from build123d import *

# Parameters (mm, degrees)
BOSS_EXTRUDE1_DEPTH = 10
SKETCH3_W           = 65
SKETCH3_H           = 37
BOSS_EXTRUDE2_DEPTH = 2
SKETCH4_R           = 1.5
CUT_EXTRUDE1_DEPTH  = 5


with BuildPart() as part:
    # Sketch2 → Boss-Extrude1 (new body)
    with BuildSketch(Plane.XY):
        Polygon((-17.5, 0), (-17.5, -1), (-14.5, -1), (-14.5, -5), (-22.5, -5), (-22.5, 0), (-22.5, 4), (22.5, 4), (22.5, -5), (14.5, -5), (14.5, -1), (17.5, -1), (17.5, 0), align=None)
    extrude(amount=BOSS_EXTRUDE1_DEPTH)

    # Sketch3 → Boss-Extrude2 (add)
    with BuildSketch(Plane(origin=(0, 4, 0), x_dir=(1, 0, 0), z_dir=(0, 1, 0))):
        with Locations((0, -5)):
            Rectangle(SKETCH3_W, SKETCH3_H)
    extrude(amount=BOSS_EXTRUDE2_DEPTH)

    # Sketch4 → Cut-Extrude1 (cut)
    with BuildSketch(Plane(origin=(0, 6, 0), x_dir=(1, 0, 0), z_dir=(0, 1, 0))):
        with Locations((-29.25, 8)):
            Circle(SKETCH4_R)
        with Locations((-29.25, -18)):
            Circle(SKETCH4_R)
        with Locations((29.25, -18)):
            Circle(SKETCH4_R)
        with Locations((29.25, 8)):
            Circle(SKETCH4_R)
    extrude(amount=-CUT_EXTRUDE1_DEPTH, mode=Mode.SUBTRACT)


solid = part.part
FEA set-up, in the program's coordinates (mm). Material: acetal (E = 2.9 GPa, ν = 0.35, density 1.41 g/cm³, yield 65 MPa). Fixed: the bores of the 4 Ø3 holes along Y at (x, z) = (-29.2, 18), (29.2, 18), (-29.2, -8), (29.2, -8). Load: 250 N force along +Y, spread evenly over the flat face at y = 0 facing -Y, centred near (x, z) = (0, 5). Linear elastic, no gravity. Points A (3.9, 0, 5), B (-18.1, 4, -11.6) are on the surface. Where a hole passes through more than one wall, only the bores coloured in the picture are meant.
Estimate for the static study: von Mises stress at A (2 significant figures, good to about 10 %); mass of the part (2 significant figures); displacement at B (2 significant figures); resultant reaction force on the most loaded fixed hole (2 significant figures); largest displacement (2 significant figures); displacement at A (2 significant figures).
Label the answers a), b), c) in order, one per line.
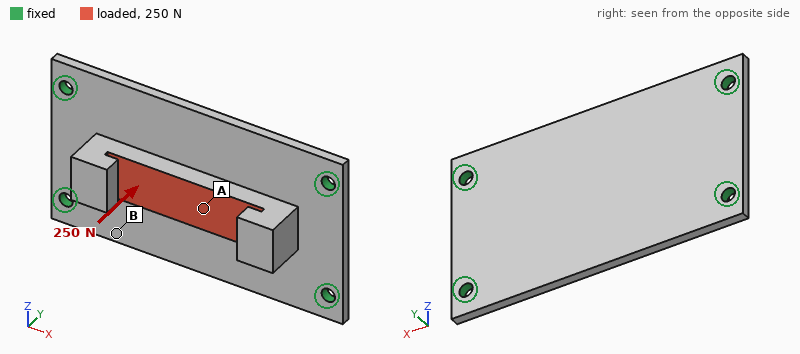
a) 21 MPa
b) 10 g
c) 0.33 mm
d) 110 N
e) 0.86 mm
f) 0.83 mm
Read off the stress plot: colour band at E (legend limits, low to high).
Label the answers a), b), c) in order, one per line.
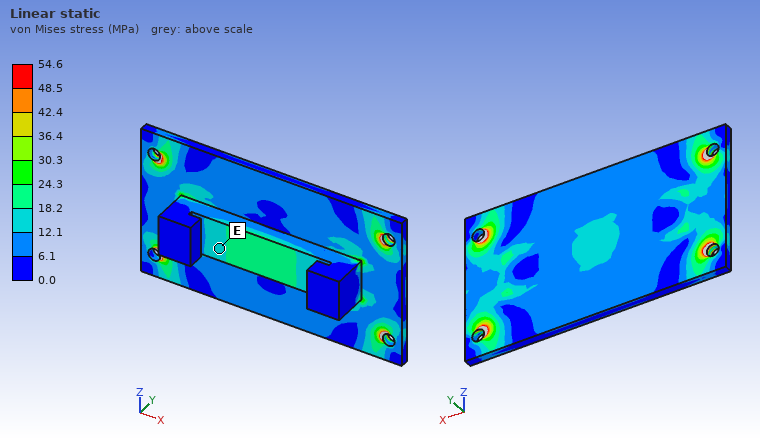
a) 12.1 to 18.2 MPa
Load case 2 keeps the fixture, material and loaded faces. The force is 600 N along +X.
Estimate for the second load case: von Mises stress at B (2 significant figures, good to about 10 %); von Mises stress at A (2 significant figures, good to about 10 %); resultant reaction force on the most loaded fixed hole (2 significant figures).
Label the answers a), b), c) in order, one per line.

a) 5.3 MPa
b) 3.1 MPa
c) 160 N
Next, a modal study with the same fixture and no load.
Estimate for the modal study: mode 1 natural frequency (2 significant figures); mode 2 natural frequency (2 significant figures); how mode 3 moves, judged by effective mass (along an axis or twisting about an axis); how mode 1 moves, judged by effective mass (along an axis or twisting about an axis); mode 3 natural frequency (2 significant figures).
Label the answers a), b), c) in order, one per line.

a) 1100 Hz
b) 1600 Hz
c) twisting about Z
d) along Y
e) 2400 Hz
